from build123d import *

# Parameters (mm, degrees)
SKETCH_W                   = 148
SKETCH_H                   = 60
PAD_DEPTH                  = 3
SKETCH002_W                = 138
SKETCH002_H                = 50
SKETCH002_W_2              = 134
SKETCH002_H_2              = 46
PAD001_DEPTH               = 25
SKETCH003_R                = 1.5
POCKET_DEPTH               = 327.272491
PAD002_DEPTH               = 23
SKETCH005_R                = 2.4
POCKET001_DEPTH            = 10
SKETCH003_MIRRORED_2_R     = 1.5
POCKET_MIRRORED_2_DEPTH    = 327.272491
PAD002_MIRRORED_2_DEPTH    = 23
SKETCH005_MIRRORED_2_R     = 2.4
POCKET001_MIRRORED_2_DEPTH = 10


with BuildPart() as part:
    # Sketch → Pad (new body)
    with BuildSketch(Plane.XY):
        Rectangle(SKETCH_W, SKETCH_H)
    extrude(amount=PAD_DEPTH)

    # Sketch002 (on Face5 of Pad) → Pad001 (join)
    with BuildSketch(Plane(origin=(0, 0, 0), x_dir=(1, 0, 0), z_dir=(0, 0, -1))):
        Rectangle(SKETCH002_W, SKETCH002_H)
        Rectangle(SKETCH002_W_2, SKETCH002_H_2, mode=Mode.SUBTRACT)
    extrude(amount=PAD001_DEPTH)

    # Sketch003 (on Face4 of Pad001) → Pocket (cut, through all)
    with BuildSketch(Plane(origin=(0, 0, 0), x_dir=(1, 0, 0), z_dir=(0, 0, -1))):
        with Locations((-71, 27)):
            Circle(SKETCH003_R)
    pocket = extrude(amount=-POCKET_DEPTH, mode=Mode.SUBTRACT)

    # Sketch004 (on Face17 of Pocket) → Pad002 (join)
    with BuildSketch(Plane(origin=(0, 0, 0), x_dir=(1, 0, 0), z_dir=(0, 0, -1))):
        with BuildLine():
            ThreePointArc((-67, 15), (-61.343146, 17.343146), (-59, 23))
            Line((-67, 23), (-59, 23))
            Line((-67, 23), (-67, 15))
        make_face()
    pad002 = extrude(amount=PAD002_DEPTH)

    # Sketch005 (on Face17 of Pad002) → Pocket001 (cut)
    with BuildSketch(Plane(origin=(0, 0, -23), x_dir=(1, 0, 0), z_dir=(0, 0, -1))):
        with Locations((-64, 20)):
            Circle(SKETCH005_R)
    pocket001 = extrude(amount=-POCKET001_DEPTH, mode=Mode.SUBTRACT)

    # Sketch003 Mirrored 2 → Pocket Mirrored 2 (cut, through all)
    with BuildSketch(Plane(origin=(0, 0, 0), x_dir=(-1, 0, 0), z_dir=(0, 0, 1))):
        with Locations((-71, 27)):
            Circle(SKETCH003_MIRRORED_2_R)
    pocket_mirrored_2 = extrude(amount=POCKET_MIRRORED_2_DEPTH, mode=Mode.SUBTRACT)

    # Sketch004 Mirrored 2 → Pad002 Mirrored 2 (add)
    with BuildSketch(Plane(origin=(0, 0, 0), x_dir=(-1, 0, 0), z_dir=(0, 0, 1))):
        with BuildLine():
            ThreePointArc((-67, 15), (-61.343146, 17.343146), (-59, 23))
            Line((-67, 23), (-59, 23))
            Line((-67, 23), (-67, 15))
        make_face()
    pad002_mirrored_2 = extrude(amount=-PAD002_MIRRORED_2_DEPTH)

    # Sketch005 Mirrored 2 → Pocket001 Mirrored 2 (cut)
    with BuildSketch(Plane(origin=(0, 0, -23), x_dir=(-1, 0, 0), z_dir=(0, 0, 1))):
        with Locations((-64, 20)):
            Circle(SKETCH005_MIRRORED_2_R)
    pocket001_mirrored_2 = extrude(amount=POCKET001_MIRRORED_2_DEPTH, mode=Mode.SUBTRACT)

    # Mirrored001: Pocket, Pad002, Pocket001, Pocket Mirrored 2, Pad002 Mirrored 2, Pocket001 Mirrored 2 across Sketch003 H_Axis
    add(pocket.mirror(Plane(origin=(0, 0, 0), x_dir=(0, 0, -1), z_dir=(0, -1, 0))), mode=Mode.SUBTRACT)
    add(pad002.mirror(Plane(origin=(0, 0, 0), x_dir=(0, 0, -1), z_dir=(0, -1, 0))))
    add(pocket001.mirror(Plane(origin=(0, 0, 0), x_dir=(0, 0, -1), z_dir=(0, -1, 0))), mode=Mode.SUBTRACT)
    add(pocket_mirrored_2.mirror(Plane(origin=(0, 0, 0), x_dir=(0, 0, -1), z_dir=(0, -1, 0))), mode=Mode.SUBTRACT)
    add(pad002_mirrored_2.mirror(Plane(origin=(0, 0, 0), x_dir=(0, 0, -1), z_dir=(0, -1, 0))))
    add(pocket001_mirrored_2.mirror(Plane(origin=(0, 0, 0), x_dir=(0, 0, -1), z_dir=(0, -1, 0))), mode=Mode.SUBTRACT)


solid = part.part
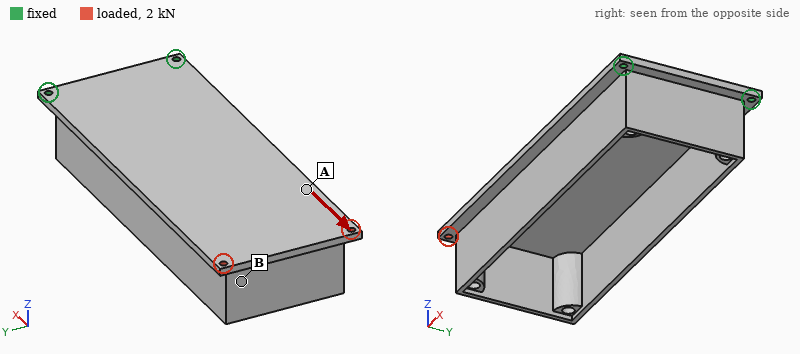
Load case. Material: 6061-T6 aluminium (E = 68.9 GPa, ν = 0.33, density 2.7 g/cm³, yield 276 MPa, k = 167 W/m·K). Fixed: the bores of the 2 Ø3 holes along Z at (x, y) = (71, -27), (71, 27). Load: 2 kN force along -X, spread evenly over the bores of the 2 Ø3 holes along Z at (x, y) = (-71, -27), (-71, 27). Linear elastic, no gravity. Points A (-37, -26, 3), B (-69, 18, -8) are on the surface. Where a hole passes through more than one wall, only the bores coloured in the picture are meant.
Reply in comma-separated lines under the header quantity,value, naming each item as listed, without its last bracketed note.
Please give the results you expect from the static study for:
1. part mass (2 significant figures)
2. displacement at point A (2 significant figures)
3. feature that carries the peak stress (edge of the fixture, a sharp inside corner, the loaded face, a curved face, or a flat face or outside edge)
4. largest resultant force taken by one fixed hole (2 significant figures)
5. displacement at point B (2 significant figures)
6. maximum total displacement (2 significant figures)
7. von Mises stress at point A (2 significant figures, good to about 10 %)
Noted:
quantity,value
part mass,130 g
displacement at point A,0.078 mm
feature that carries the peak stress,the loaded face
largest resultant force taken by one fixed hole,1.1 kN
displacement at point B,0.12 mm
maximum total displacement,0.13 mm
von Mises stress at point A,13 MPa
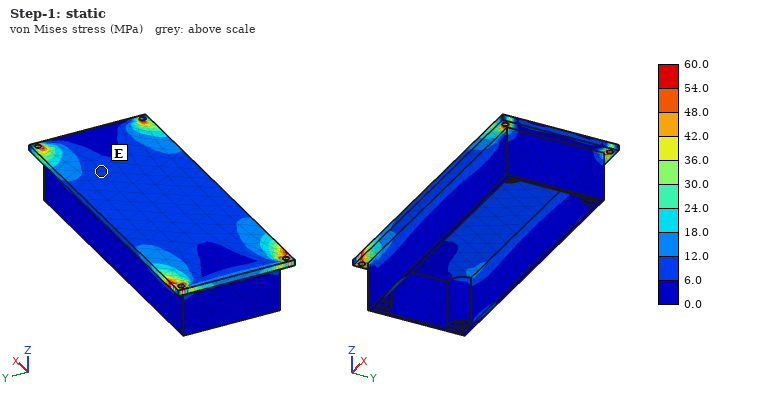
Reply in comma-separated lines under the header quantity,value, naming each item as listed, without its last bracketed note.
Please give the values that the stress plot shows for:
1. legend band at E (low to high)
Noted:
quantity,value
legend band at E,6.0 to 12.0 MPa
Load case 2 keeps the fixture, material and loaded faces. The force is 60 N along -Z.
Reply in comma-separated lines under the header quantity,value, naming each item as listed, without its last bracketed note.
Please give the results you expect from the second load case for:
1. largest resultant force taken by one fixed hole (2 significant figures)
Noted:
quantity,value
largest resultant force taken by one fixed hole,54 N
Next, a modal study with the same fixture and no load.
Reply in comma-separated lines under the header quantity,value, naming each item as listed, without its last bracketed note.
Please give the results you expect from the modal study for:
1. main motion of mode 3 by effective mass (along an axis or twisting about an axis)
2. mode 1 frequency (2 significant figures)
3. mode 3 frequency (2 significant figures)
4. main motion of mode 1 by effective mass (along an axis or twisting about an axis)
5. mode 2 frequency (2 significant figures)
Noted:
quantity,value
main motion of mode 3 by effective mass,along Y
mode 1 frequency,150 Hz
mode 3 frequency,1500 Hz
main motion of mode 1 by effective mass,along Z
mode 2 frequency,490 Hz
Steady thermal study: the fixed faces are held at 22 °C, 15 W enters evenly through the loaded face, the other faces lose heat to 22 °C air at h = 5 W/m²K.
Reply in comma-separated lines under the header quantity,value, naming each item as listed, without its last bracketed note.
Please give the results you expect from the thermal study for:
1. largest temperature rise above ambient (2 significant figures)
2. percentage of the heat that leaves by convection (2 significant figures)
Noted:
quantity,value
largest temperature rise above ambient,54 K
percentage of the heat that leaves by convection,28 %
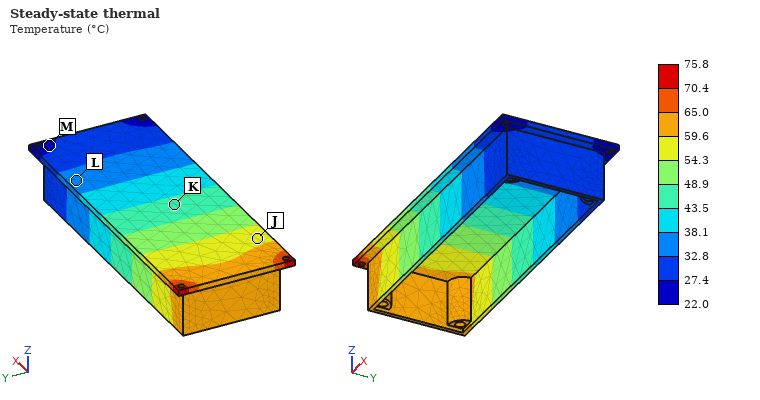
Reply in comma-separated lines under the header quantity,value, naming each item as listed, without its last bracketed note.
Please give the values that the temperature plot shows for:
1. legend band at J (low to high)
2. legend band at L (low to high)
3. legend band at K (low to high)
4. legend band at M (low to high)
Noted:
quantity,value
legend band at J,54.3 to 59.6 °C
legend band at L,32.8 to 38.1 °C
legend band at K,43.5 to 48.9 °C
legend band at M,22.0 to 27.4 °C
